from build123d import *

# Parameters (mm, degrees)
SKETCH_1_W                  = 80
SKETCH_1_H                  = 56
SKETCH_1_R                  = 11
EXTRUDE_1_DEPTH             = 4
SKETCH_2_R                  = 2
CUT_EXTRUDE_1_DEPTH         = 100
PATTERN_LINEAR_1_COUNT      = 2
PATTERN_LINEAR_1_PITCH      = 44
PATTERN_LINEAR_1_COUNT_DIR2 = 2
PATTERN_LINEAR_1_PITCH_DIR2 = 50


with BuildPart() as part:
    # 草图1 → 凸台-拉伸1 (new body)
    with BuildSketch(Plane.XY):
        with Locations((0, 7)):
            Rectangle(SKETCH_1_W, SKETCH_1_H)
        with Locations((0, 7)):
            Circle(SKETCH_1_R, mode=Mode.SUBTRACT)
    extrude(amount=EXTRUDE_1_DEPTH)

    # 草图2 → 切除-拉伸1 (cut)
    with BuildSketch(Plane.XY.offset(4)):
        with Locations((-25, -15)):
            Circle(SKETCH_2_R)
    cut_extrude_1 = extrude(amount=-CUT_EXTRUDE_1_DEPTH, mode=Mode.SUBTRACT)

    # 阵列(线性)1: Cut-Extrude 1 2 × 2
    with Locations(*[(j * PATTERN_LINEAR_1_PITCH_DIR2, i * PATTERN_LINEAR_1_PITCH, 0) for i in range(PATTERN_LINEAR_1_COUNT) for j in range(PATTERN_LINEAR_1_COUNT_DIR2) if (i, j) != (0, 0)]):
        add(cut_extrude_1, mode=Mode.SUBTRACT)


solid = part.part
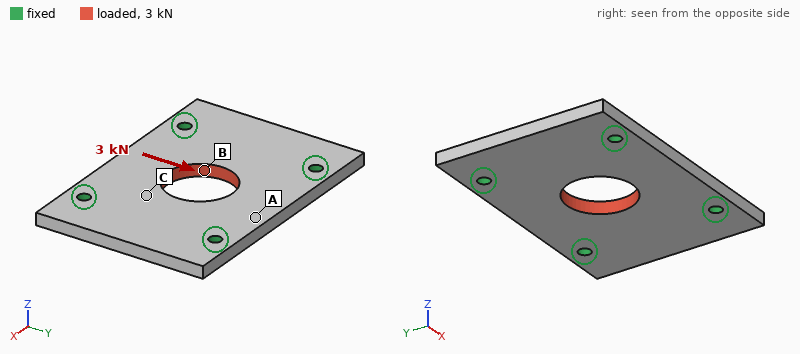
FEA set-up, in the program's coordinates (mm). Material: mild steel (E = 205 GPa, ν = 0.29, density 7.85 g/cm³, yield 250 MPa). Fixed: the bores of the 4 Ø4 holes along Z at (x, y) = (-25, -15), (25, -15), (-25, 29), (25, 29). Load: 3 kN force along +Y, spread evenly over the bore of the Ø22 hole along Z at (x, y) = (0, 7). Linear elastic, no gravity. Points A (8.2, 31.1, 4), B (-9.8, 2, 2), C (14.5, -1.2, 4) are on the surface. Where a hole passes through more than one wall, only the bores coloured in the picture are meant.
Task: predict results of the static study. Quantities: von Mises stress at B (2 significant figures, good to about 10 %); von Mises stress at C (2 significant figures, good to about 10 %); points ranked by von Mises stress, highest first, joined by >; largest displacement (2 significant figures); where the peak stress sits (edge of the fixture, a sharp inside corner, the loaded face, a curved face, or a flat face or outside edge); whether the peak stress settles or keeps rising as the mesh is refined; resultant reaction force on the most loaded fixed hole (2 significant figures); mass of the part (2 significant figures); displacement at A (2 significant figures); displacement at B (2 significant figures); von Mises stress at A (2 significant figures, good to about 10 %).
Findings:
22 MPa
13 MPa
B > C > A
2.7 µm
edge of the fixture
keeps rising
840 N
130 g
1.9 µm
2.0 µm
6.5 MPa
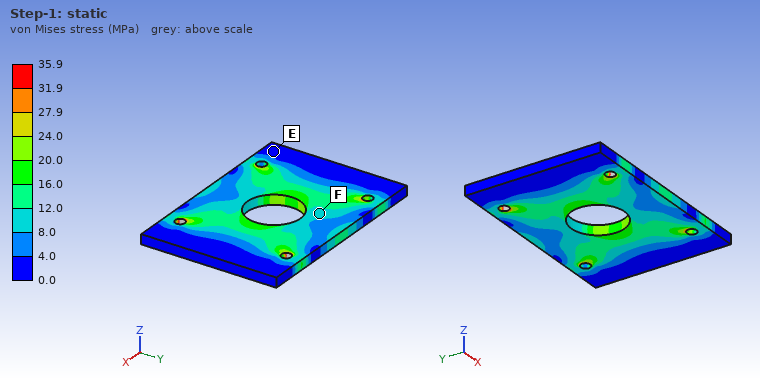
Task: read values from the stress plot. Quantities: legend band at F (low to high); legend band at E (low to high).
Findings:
8.0 to 12.0 MPa
0.0 to 4.0 MPa
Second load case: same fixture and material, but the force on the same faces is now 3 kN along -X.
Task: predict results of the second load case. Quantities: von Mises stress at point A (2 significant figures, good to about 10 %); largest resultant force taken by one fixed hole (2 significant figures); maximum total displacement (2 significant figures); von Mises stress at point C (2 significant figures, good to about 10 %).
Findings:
4.4 MPa
770 N
1.8 µm
9.6 MPa
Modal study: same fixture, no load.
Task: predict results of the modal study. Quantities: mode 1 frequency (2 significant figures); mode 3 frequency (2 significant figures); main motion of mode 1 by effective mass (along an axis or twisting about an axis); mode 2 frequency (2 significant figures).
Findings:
6900 Hz
8600 Hz
along Z
8400 Hz
